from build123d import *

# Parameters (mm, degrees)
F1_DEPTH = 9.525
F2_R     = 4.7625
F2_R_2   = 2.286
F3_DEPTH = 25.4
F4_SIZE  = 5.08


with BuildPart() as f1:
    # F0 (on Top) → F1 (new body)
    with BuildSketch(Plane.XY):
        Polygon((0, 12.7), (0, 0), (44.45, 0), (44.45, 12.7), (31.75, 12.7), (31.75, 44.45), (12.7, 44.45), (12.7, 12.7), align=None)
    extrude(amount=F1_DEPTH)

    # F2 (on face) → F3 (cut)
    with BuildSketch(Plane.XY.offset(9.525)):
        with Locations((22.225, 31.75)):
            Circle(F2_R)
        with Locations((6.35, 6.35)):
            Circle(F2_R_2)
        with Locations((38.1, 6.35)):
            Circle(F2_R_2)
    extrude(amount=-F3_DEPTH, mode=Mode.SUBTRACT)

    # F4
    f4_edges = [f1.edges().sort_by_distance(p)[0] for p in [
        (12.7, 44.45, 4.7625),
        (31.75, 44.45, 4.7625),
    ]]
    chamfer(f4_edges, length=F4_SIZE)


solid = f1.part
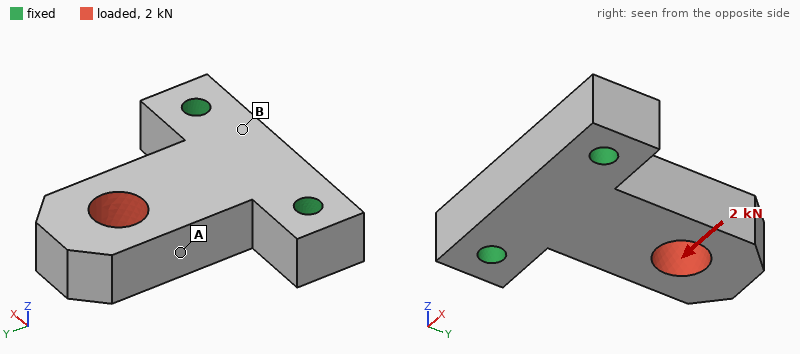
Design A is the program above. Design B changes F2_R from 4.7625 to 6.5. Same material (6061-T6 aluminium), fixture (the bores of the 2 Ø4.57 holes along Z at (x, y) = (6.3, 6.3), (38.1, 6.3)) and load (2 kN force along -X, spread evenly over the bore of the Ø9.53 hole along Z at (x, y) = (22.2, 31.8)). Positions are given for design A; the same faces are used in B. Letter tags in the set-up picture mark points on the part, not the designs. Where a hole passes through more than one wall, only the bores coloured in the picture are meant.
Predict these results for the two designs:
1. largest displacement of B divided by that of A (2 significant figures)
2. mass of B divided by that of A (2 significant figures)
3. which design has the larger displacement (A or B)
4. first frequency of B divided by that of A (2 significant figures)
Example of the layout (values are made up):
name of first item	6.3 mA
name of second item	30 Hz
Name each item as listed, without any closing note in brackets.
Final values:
largest displacement of B divided by that of A	1.4
mass of B divided by that of A	0.94
which design has the larger displacement	B
first frequency of B divided by that of A	1.1
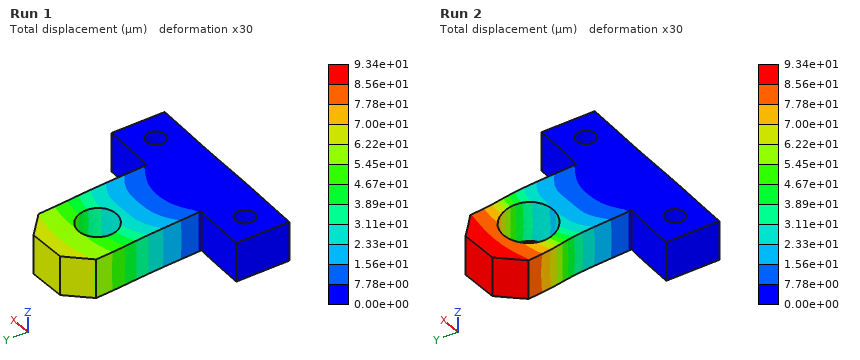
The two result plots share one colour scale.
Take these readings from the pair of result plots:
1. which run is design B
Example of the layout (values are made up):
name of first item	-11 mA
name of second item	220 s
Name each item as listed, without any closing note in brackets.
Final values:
which run is design B	Run 2
